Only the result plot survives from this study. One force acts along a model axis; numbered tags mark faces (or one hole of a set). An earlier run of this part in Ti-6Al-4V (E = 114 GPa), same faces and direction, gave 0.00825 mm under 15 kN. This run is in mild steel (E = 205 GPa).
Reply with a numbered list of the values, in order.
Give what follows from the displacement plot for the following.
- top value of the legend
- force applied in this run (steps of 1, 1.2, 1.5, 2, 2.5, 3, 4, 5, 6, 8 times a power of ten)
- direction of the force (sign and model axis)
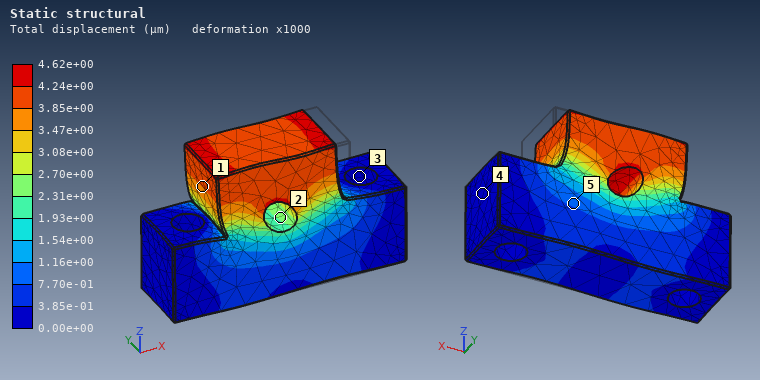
1. 4.62e+00 µm
2. 15 kN
3. -X
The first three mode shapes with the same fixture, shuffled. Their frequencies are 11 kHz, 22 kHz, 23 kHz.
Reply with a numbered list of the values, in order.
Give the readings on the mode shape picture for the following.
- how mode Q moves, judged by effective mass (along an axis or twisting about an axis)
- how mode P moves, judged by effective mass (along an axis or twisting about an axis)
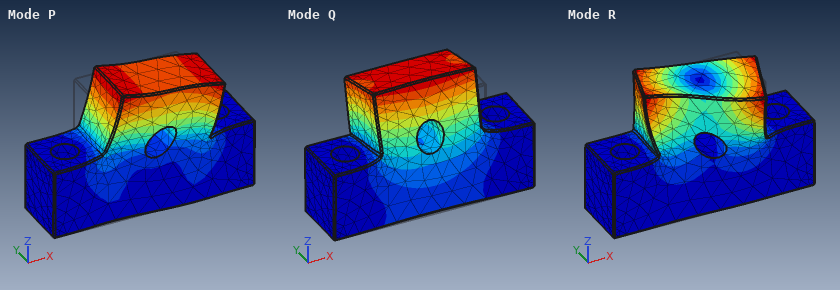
1. along Y
2. along X
